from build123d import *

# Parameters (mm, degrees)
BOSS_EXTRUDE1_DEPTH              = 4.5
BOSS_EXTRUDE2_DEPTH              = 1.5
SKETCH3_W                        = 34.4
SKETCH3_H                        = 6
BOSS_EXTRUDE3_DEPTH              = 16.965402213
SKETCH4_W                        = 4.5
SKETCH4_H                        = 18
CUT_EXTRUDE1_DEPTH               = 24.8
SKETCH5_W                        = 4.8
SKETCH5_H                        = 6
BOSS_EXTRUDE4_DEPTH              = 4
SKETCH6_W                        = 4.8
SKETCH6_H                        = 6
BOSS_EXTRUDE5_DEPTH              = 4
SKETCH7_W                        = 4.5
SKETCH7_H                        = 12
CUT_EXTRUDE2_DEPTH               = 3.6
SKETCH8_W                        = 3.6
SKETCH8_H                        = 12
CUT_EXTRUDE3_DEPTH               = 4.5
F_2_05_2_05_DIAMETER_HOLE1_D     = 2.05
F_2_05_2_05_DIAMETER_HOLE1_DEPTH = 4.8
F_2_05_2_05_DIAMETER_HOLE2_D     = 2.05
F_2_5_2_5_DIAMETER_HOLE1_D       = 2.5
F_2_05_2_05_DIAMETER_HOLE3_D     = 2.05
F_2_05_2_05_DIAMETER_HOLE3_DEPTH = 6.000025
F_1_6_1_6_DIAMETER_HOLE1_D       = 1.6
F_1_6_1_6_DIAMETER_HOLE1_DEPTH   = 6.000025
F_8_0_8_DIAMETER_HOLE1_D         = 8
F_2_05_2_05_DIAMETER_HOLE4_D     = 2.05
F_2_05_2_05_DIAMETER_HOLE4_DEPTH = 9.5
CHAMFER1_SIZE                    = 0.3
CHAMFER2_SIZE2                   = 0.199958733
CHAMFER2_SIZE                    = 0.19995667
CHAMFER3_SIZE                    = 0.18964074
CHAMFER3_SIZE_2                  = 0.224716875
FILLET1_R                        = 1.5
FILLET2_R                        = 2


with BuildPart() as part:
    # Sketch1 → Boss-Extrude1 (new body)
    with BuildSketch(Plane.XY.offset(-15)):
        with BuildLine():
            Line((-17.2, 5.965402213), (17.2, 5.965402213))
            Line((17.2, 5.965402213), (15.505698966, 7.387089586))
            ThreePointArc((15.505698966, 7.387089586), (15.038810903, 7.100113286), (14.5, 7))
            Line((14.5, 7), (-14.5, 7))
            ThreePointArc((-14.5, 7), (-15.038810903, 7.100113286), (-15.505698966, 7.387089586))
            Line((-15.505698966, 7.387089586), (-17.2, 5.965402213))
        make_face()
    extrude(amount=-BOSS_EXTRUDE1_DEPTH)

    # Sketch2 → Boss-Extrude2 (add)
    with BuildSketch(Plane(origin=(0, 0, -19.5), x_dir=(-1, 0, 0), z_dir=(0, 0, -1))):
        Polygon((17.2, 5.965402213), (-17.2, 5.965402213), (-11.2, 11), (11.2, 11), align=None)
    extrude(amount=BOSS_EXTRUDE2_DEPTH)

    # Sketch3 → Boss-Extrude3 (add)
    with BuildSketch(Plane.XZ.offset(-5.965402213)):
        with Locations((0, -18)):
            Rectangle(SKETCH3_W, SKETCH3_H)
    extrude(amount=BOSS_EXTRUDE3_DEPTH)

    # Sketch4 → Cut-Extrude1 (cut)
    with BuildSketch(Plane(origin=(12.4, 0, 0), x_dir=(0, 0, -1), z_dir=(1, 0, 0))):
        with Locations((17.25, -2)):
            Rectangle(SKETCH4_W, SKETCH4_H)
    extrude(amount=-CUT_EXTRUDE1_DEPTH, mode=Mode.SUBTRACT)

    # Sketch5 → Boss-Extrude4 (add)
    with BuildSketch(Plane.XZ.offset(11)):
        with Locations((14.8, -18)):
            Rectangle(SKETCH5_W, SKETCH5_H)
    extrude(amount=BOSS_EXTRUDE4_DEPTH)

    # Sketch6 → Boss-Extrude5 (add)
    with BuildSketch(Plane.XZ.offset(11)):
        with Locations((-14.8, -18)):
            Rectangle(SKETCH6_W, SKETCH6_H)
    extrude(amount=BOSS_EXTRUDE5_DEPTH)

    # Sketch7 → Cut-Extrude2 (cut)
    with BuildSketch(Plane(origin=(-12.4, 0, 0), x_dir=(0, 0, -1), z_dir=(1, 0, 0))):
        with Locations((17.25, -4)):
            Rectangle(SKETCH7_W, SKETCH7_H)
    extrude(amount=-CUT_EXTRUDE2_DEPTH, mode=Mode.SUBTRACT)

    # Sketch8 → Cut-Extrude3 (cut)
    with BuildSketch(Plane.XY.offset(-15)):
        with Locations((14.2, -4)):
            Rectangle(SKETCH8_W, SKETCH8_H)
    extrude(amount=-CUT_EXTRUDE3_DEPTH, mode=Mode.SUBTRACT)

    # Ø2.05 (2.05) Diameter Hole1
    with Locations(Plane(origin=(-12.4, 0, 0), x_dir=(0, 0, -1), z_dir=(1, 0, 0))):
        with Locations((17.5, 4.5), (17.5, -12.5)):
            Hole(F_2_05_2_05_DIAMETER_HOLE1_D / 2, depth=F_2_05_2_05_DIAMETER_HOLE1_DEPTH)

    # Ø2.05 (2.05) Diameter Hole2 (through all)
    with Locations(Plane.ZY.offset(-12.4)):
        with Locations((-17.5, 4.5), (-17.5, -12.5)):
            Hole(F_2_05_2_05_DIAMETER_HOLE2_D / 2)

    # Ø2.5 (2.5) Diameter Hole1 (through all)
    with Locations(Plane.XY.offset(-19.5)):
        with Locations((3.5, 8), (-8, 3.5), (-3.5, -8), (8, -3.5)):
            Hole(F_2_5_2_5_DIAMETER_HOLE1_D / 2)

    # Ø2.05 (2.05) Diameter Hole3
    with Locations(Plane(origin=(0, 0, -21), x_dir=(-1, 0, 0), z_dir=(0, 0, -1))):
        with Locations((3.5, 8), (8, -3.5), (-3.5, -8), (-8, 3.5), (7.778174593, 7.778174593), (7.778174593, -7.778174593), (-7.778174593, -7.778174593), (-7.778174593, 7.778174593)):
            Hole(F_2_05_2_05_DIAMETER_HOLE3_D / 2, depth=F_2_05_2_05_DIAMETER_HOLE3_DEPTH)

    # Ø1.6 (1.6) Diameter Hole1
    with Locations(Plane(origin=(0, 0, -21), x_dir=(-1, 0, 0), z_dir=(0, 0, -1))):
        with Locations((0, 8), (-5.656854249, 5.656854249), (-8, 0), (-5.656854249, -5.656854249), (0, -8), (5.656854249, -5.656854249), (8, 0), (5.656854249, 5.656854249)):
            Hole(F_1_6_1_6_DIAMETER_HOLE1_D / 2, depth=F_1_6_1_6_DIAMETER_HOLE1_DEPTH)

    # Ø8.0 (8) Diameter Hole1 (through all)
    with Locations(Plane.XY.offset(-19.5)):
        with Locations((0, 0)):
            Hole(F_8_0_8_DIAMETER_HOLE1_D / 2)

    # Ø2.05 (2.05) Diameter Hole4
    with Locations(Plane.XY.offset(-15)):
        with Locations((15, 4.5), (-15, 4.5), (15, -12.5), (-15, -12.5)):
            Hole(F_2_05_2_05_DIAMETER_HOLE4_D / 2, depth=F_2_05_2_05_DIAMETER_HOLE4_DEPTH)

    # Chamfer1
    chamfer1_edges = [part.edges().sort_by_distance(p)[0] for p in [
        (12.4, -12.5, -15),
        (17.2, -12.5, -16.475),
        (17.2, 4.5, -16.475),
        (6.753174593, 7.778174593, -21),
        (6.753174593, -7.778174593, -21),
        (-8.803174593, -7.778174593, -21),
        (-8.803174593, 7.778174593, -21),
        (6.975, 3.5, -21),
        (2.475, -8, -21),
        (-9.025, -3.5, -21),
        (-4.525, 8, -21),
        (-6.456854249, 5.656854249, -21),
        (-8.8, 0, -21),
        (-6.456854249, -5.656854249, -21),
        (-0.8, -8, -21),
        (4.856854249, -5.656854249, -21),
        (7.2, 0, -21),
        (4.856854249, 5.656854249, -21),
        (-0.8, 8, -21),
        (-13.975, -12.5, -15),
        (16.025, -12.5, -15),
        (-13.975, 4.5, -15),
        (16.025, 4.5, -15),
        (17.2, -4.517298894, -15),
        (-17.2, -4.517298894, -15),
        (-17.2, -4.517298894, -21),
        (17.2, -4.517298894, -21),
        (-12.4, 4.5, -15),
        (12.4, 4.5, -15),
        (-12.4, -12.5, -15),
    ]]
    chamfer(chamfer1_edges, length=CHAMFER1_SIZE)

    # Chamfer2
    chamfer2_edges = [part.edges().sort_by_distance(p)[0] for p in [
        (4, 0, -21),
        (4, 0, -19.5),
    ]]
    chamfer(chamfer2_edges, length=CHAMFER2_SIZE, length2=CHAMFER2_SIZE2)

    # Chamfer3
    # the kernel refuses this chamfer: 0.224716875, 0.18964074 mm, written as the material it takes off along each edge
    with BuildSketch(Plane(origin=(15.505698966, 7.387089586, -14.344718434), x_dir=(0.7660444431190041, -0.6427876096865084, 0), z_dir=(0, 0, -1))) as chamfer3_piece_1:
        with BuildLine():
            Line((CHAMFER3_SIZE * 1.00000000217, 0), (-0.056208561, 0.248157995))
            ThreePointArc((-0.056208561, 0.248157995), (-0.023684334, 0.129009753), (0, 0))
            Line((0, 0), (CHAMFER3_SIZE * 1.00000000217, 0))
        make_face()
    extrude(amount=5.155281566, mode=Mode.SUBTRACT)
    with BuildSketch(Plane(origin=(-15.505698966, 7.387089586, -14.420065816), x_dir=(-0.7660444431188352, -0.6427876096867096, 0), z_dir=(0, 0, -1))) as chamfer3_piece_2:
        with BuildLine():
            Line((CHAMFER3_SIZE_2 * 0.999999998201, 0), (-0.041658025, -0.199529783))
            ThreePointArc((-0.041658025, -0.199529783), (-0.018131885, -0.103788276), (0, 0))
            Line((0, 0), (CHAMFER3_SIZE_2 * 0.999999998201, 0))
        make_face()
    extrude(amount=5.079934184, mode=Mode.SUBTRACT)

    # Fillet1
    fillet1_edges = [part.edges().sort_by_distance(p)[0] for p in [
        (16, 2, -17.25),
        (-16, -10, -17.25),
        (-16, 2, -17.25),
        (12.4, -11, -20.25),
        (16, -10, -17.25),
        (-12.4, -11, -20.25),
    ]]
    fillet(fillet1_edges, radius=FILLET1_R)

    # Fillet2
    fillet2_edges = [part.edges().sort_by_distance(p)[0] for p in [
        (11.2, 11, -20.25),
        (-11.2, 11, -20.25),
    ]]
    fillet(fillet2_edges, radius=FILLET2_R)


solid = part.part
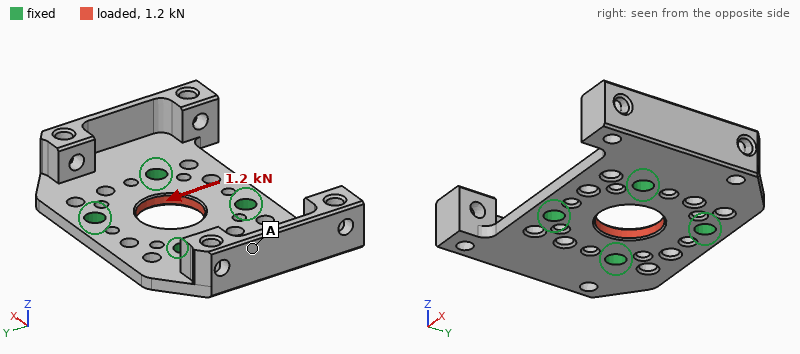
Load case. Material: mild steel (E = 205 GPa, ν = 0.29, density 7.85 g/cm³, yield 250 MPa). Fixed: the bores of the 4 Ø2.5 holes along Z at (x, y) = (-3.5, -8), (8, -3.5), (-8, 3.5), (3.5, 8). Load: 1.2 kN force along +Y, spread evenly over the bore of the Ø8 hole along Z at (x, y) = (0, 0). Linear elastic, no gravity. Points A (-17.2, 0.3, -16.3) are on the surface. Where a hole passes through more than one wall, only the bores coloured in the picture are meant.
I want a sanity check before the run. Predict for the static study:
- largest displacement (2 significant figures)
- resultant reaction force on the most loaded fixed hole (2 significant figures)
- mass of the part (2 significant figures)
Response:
1.6 µm
350 N
11 g
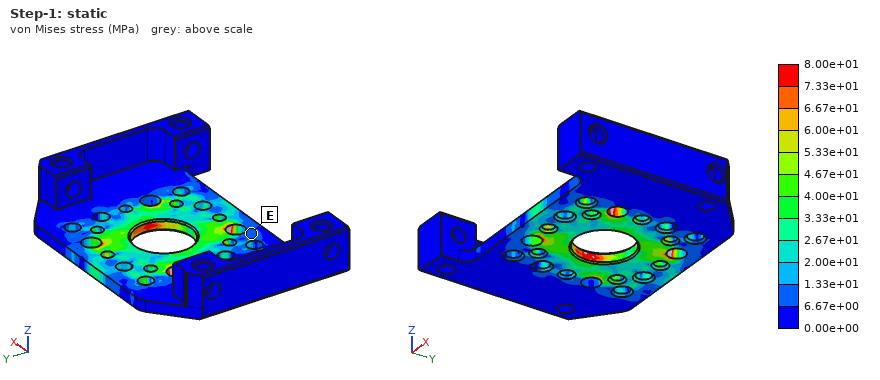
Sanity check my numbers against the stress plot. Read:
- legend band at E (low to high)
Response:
6.67e+00 to 1.33e+01 MPa
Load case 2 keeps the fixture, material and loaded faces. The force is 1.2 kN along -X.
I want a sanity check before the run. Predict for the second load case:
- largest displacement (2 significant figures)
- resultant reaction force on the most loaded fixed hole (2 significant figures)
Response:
1.5 µm
360 N
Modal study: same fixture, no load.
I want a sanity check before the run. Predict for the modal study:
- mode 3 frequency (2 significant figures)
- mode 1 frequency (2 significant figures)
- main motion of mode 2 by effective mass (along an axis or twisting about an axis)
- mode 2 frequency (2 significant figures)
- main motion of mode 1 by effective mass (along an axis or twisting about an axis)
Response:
7700 Hz
5000 Hz
along Z
6800 Hz
along Z
